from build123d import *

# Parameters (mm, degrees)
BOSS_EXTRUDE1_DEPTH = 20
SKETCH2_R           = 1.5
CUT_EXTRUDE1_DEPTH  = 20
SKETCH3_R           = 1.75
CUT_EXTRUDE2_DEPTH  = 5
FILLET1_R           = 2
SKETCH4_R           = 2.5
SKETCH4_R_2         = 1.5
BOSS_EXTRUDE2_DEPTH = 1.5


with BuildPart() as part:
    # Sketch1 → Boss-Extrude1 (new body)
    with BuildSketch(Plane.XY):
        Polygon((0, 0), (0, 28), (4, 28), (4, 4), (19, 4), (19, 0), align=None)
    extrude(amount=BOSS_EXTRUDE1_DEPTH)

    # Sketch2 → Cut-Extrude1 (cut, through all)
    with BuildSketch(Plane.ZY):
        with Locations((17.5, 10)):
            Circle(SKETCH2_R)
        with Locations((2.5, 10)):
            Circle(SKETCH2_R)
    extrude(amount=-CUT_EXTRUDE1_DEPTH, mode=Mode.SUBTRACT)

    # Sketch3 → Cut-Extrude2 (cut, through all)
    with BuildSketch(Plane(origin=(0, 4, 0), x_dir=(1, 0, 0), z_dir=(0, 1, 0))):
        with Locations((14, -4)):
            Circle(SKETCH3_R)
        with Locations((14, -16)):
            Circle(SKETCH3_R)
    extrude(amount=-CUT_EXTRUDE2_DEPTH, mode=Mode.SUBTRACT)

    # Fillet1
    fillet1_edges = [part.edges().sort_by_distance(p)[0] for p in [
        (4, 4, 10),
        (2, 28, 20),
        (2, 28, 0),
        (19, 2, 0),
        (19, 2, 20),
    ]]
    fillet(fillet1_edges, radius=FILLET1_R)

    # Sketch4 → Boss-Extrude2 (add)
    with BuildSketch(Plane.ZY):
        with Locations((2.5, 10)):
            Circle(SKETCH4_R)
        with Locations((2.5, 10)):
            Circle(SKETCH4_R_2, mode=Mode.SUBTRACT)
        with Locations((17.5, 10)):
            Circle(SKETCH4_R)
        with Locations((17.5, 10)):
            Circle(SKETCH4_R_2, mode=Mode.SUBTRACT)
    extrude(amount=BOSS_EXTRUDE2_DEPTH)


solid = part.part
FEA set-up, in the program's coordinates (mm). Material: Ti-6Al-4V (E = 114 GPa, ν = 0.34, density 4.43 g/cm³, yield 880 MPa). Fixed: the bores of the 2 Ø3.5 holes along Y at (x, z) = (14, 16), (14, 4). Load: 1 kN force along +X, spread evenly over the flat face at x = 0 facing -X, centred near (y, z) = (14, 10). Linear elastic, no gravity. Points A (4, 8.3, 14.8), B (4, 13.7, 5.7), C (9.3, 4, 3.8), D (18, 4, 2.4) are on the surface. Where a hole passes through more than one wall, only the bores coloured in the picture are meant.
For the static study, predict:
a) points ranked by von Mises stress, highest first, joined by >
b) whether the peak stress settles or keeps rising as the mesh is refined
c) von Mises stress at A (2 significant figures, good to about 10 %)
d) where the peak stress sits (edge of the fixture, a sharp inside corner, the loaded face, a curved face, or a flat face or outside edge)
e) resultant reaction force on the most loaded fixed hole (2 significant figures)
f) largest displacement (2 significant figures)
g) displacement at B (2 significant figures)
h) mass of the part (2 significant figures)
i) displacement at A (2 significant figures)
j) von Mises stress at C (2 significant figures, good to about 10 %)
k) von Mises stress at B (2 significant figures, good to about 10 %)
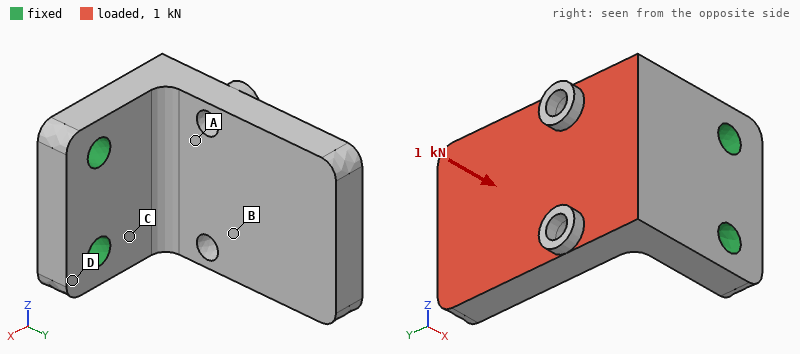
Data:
C > A > B > D
keeps rising
160 MPa
edge of the fixture
520 N
0.40 mm
0.15 mm
15 g
0.079 mm
250 MPa
79 MPa
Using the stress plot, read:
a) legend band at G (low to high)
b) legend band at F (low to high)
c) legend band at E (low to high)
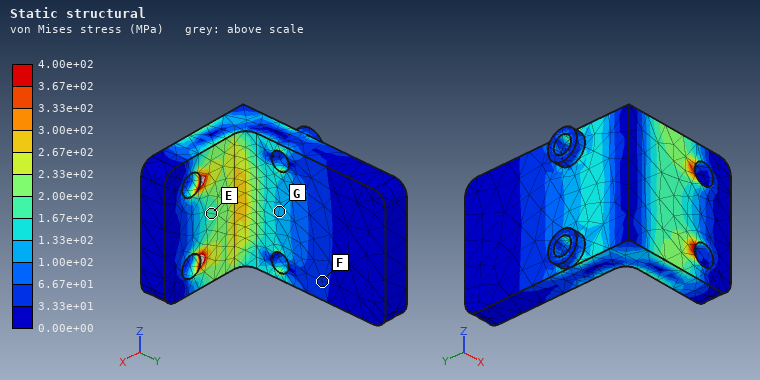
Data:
1.00e+02 to 1.33e+02 MPa
3.33e+01 to 6.67e+01 MPa
1.67e+02 to 2.00e+02 MPa
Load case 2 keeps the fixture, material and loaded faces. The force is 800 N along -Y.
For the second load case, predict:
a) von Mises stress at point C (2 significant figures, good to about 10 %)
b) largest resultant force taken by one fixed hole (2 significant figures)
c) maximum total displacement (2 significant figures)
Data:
140 MPa
400 N
0.17 mm
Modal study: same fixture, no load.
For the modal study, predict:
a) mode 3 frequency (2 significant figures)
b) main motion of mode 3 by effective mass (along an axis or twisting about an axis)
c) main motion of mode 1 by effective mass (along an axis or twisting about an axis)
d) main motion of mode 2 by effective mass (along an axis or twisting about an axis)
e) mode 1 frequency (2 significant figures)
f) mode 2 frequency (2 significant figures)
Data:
11 kHz
along Y
along X
along Z
3100 Hz
5700 Hz
